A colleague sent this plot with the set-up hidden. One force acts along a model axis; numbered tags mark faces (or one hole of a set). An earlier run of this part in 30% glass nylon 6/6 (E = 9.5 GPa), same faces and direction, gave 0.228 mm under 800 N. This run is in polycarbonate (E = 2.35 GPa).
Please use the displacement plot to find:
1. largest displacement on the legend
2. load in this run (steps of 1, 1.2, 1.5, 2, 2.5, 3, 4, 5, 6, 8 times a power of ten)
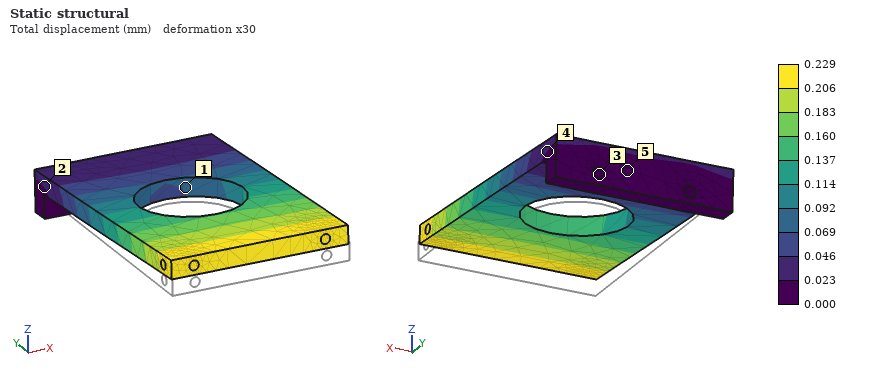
0.229 mm
200 N
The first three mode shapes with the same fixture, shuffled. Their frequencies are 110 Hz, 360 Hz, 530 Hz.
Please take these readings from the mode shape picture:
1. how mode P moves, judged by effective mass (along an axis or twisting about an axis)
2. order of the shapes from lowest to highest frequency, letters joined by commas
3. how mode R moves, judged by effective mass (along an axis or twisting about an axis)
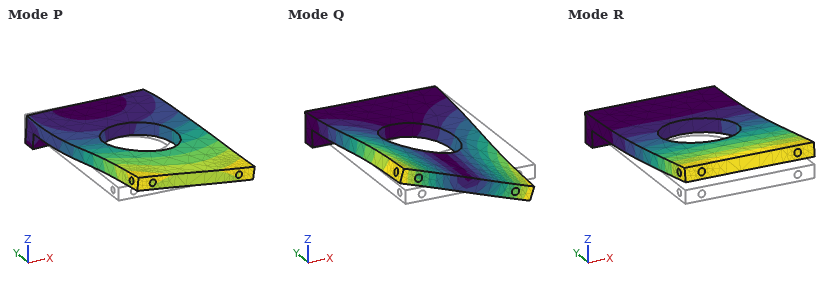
along X
R, Q, P
along Z
